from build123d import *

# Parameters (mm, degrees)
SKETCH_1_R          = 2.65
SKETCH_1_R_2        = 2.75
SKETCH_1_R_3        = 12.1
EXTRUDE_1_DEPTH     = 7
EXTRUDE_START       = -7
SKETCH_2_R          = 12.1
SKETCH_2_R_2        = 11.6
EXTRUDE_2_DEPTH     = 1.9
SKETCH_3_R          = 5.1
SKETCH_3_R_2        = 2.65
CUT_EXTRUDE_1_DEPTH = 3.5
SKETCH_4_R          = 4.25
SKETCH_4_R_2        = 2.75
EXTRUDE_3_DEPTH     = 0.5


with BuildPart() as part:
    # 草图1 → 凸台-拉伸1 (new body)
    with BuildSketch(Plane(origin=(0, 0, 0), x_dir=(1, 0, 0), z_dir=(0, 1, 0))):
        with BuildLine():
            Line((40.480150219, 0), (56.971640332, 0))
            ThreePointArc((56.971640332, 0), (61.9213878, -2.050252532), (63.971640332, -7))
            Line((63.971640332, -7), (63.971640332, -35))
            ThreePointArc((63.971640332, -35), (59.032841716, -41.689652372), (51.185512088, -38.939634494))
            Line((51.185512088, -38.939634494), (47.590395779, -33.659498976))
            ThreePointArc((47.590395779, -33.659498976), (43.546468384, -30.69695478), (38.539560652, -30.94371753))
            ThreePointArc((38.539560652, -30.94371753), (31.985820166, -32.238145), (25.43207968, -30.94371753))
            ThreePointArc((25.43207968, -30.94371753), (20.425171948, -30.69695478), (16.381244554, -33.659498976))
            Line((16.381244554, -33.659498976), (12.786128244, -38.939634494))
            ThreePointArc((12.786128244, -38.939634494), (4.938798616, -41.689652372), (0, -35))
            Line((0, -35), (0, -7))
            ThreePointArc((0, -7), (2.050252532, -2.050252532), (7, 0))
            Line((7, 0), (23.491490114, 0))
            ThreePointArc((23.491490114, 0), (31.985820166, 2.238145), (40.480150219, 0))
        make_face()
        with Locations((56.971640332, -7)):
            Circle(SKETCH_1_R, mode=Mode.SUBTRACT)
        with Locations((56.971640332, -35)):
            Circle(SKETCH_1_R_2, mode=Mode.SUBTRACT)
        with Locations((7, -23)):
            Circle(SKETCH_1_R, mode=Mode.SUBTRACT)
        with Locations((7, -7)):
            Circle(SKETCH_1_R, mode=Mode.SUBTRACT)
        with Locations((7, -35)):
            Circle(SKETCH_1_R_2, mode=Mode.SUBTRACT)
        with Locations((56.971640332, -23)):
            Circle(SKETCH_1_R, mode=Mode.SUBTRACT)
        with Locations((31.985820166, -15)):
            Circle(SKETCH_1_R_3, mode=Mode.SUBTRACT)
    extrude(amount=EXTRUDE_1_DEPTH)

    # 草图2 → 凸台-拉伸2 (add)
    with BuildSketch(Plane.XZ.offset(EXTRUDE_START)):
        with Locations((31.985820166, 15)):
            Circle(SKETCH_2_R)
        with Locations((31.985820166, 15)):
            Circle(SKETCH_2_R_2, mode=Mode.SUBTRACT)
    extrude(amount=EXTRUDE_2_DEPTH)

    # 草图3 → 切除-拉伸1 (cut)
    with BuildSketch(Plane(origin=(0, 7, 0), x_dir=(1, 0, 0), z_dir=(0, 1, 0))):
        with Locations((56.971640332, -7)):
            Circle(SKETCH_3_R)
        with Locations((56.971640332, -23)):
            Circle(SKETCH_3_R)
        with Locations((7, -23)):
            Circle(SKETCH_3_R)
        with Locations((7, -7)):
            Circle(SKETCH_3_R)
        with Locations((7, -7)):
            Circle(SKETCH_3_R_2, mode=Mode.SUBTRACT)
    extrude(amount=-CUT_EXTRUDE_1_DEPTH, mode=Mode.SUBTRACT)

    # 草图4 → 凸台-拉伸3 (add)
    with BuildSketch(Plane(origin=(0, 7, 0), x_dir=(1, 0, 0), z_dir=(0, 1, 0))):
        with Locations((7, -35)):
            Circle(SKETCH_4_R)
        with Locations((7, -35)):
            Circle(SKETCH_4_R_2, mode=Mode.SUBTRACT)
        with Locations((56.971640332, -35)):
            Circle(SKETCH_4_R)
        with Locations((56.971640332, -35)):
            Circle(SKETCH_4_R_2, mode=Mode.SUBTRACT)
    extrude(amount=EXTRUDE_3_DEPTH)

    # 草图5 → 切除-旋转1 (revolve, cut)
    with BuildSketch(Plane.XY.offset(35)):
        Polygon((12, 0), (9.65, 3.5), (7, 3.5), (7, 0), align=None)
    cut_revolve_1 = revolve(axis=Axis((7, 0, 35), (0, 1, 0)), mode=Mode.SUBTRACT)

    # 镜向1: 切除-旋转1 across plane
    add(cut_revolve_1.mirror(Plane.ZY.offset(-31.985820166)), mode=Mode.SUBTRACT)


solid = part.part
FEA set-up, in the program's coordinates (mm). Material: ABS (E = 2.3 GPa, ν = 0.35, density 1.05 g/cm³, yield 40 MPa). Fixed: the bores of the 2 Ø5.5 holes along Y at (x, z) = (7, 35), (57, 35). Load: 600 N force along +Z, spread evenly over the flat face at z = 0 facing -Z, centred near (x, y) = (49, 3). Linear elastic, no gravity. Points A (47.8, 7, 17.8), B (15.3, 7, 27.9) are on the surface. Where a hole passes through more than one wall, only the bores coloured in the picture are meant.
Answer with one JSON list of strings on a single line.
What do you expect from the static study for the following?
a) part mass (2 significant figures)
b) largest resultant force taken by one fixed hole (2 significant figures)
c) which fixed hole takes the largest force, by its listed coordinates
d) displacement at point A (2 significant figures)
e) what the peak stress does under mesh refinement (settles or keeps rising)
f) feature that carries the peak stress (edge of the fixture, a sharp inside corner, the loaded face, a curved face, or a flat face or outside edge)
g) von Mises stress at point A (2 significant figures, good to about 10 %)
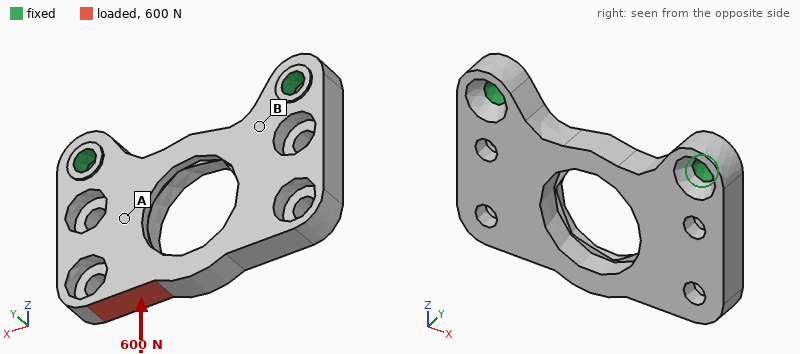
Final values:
["11 g", "540 N", "(57, 35)", "0.10 mm", "keeps rising", "edge of the fixture", "7.9 MPa"]
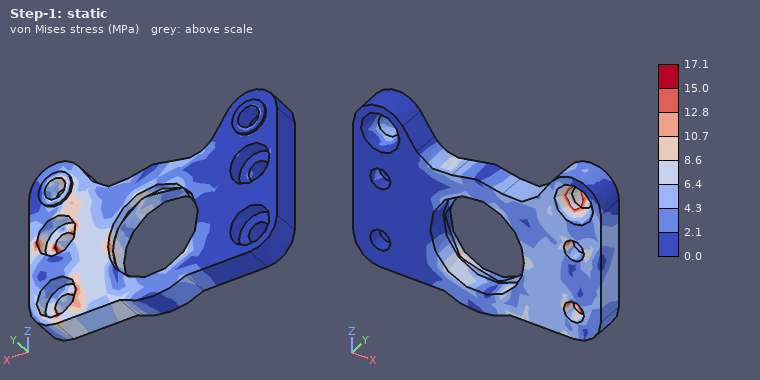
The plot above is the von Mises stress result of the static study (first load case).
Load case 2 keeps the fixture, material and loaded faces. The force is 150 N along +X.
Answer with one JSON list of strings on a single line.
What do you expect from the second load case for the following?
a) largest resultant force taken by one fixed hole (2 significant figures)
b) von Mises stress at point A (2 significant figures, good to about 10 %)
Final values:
["110 N", "1.9 MPa"]
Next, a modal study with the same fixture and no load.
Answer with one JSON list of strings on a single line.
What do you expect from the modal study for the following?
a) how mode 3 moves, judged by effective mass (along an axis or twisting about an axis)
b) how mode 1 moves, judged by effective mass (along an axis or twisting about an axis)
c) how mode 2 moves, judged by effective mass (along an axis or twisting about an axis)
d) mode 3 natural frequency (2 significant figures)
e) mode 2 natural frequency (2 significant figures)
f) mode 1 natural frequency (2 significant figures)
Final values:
["along X", "along Y", "twisting about Z", "2600 Hz", "1700 Hz", "880 Hz"]
